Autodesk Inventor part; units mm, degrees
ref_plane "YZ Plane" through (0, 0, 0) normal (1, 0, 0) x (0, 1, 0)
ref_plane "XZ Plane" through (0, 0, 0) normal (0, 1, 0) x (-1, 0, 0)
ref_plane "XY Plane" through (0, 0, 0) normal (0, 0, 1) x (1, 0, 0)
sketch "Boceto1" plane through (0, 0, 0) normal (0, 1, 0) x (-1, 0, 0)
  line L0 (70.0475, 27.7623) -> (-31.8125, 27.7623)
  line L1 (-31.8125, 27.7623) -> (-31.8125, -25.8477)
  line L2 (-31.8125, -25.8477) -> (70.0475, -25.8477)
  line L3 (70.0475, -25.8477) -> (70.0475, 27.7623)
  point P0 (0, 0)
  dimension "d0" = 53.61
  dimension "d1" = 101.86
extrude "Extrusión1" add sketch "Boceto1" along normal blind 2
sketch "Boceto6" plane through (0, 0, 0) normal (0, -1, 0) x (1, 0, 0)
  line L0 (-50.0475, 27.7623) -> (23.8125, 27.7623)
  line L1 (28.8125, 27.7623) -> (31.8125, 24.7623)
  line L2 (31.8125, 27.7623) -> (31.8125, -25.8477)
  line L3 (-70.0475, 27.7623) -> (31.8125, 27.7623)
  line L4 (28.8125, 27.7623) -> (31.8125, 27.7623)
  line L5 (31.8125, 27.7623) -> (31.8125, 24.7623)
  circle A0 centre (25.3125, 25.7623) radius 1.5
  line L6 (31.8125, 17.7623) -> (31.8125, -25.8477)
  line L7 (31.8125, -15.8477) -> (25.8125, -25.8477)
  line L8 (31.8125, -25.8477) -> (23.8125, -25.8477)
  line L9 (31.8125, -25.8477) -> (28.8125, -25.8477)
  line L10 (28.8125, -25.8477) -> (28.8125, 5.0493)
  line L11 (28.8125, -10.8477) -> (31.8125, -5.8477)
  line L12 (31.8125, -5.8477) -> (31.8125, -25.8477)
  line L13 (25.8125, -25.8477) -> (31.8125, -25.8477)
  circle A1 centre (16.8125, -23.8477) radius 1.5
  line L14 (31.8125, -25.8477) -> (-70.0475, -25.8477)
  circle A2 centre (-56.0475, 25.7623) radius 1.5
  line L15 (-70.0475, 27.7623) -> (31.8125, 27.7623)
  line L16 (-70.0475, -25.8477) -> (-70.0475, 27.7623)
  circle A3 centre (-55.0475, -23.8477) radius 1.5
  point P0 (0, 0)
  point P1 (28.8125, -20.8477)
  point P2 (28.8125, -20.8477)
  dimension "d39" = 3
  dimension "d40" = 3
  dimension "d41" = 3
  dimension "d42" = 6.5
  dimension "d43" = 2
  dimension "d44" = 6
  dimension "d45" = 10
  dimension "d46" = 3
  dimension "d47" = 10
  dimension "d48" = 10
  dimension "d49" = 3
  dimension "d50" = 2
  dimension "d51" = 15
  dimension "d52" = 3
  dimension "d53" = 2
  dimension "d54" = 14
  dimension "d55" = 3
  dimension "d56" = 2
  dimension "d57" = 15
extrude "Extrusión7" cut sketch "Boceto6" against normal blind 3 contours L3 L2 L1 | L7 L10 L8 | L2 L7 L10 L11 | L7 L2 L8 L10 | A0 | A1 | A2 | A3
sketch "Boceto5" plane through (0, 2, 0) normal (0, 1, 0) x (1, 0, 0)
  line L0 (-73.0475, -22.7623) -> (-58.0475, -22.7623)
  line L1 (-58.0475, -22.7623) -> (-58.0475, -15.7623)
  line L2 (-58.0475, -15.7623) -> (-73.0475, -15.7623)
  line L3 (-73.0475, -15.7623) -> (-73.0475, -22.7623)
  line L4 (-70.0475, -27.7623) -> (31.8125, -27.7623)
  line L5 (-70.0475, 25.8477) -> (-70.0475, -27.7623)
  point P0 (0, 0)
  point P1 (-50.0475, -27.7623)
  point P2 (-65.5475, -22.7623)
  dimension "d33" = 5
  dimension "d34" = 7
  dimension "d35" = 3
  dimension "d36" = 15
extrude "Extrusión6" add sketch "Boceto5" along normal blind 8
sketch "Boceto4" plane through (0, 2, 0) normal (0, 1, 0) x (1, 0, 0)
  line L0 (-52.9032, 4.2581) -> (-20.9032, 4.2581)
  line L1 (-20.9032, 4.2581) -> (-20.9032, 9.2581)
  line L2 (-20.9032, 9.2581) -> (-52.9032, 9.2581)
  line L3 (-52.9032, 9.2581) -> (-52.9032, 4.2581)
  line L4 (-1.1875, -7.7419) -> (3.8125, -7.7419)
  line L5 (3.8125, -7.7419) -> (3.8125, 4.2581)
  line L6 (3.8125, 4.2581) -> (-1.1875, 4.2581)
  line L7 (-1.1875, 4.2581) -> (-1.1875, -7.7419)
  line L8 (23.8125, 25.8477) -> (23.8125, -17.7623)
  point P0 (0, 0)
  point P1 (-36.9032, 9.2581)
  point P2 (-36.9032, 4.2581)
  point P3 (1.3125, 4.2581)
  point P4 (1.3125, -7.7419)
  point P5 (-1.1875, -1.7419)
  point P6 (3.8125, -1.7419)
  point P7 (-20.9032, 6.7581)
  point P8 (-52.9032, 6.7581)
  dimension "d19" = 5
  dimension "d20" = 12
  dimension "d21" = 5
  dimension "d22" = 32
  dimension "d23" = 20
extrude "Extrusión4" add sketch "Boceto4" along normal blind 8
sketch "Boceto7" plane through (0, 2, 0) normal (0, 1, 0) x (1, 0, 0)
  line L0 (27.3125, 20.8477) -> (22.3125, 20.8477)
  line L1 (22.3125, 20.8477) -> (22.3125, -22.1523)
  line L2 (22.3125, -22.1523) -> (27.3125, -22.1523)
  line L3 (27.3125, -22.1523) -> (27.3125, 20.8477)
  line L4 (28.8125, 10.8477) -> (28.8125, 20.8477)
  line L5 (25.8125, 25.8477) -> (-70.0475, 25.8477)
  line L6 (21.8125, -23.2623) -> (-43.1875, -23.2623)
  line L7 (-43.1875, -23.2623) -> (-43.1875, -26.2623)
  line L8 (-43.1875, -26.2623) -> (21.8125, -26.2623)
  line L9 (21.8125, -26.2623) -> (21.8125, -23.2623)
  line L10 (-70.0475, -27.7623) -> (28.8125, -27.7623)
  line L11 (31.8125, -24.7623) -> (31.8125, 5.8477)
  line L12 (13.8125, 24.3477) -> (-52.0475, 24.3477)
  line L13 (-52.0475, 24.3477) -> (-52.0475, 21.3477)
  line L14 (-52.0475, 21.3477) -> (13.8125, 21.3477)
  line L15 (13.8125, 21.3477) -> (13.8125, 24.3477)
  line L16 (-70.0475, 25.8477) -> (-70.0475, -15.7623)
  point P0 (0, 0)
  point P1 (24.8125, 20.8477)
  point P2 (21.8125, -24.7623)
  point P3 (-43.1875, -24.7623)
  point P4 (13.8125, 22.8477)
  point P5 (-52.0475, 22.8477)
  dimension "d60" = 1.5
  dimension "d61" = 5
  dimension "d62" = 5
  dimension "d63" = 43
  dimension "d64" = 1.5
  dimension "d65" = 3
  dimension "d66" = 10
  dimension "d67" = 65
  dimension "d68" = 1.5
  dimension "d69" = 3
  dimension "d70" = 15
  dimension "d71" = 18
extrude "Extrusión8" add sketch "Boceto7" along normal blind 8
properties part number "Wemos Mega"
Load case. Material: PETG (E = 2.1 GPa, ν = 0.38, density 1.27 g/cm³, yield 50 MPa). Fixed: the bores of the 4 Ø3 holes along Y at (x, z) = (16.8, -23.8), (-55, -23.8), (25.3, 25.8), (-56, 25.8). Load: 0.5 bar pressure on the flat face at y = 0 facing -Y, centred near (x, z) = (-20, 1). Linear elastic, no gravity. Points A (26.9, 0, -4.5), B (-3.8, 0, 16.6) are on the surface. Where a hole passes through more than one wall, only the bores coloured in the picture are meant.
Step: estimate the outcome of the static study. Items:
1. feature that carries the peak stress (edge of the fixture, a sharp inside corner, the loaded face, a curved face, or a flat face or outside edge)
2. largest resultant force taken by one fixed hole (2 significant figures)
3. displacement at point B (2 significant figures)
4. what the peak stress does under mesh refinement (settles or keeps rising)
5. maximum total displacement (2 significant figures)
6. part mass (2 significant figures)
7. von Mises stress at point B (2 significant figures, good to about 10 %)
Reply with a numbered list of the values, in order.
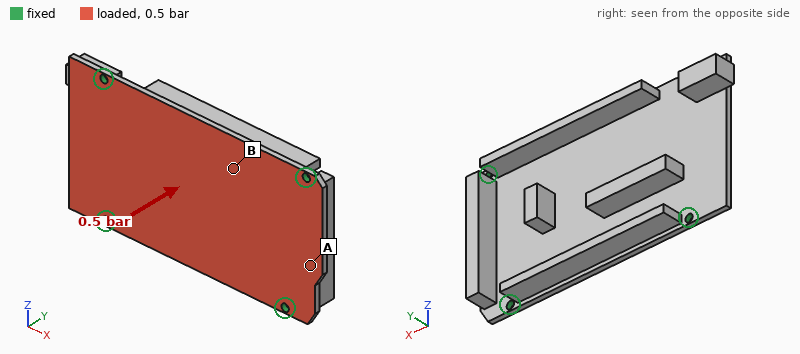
1. edge of the fixture
2. 84 N
3. 0.86 mm
4. keeps rising
5. 1.4 mm
6. 23 g
7. 5.7 MPa
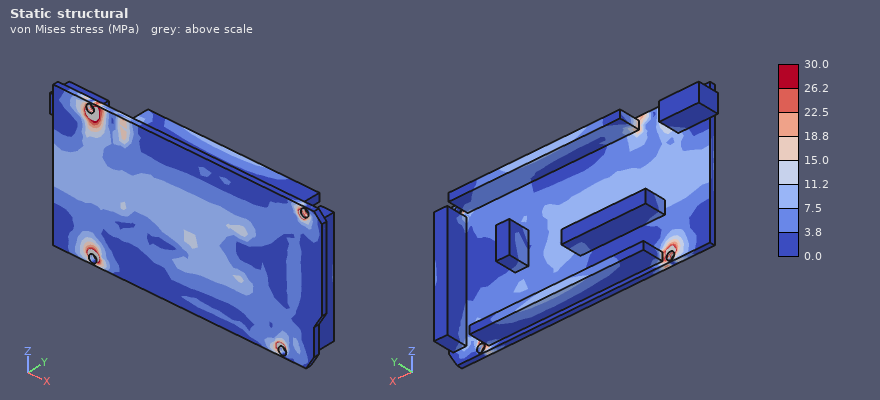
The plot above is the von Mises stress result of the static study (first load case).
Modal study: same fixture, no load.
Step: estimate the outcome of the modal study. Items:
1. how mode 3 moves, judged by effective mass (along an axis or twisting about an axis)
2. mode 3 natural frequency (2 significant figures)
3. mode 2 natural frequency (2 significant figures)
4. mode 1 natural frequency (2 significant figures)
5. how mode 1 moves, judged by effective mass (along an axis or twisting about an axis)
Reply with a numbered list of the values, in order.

1. twisting about X
2. 1000 Hz
3. 790 Hz
4. 610 Hz
5. along Y
